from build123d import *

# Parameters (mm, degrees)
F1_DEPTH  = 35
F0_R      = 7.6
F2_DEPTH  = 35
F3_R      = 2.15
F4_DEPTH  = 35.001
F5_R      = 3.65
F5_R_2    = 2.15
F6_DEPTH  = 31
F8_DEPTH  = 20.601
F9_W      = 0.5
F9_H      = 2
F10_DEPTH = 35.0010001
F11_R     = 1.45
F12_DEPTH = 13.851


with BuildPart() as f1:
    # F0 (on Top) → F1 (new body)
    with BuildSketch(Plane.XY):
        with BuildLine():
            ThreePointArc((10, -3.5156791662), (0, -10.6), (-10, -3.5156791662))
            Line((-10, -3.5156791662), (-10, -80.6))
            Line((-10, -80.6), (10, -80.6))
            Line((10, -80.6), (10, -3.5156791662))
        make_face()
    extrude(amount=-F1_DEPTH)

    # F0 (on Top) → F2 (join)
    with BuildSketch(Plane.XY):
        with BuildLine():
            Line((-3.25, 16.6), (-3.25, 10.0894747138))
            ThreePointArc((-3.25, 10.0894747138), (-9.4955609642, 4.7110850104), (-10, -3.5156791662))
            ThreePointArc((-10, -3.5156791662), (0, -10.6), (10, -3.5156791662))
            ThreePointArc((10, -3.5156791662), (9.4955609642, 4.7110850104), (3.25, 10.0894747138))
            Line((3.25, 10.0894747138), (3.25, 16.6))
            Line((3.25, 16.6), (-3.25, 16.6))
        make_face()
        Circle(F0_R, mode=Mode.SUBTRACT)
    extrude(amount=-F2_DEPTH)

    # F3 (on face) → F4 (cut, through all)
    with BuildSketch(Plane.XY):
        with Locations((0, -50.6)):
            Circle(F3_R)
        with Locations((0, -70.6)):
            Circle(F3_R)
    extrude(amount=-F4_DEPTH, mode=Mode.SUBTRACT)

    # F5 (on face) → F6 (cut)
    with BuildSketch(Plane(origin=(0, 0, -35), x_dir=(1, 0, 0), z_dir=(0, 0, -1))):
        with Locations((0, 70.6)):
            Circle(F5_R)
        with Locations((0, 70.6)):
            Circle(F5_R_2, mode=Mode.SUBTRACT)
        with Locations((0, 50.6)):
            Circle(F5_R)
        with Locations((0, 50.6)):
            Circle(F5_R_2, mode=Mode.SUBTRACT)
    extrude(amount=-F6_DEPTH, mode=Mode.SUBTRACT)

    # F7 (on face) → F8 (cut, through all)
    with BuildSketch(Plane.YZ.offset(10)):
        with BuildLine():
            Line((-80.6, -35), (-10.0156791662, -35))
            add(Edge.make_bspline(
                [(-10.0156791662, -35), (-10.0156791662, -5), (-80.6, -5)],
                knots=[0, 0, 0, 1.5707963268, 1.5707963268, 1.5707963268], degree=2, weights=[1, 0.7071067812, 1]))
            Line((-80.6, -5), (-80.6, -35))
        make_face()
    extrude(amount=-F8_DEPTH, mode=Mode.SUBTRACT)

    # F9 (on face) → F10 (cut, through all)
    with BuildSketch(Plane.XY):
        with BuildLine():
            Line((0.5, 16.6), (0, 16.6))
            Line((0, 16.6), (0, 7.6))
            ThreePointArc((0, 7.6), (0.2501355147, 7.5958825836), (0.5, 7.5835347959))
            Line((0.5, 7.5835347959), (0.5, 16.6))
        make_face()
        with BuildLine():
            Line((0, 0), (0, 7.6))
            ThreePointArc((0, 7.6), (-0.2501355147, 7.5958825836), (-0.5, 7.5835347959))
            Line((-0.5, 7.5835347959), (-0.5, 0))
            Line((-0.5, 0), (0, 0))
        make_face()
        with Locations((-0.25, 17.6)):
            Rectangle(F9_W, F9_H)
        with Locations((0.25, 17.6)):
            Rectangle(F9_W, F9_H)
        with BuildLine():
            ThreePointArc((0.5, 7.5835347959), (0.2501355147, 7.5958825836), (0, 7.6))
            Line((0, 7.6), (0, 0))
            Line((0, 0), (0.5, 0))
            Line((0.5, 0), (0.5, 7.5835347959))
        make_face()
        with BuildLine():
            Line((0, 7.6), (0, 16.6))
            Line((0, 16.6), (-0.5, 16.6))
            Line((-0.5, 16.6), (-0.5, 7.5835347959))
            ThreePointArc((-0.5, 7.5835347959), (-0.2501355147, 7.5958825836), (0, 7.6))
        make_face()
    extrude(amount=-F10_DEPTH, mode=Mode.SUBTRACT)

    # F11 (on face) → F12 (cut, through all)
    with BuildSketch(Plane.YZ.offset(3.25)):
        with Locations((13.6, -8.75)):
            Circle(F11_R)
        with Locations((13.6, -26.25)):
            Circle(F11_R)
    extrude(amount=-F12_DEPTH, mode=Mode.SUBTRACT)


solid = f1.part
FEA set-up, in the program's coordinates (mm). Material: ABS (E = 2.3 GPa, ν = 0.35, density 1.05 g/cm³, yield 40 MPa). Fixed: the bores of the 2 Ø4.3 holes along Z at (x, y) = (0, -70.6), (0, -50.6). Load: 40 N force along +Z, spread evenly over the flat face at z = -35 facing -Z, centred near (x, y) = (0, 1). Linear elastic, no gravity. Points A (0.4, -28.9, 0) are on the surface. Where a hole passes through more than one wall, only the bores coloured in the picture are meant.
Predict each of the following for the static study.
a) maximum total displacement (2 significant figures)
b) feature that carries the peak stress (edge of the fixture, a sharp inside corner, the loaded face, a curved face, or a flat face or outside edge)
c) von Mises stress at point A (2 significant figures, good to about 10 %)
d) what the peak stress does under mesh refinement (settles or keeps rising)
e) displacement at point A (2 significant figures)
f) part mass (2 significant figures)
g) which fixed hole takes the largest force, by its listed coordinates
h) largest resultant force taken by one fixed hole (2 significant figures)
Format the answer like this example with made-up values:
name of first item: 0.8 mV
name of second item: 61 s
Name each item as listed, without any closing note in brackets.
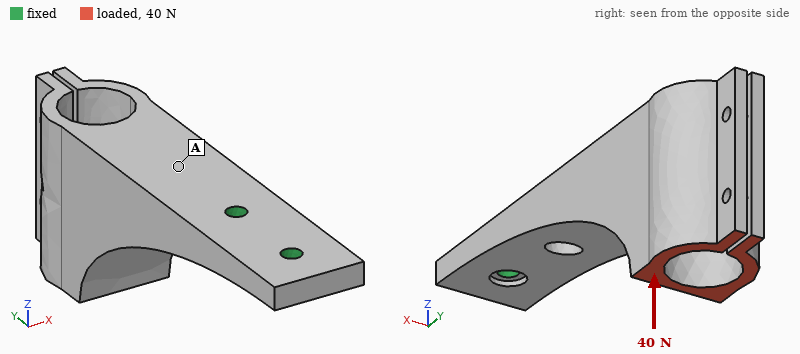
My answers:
maximum total displacement: 1.2 mm
feature that carries the peak stress: edge of the fixture
von Mises stress at point A: 2.0 MPa
what the peak stress does under mesh refinement: keeps rising
displacement at point A: 0.30 mm
part mass: 25 g
which fixed hole takes the largest force, by its listed coordinates: (0, -50.6)
largest resultant force taken by one fixed hole: 140 N
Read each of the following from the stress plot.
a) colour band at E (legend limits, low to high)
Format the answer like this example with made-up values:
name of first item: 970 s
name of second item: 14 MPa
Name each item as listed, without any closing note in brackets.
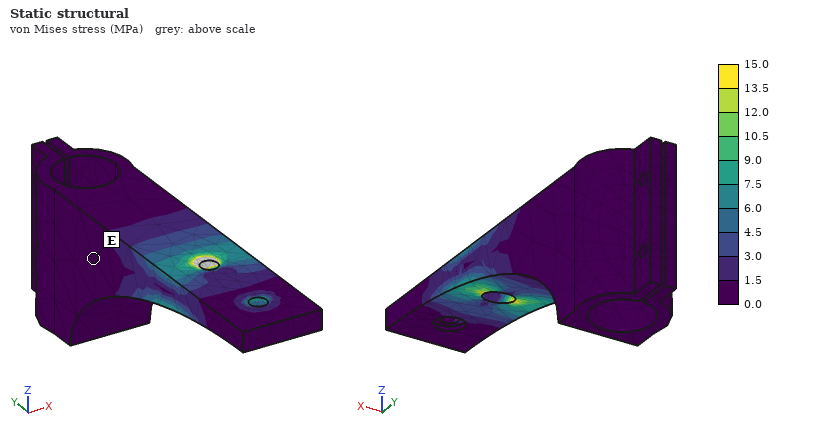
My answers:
colour band at E: 0.0 to 1.5 MPa
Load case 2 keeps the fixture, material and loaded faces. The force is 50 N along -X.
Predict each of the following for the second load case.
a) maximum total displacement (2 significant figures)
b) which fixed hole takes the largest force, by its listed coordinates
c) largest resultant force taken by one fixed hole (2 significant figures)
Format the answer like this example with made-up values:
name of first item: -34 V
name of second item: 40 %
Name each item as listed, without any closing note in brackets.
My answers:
maximum total displacement: 1.1 mm
which fixed hole takes the largest force, by its listed coordinates: (0, -50.6)
largest resultant force taken by one fixed hole: 140 N
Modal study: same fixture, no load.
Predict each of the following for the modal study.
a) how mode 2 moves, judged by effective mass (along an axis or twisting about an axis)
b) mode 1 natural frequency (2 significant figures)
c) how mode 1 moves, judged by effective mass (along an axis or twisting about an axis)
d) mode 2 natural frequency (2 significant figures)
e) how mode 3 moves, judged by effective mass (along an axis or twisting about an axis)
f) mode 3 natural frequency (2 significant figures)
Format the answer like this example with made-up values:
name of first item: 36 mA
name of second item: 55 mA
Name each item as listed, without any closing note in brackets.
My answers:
how mode 2 moves, judged by effective mass: along X
mode 1 natural frequency: 300 Hz
how mode 1 moves, judged by effective mass: along Z
mode 2 natural frequency: 510 Hz
how mode 3 moves, judged by effective mass: twisting about Y
mode 3 natural frequency: 1100 Hz
